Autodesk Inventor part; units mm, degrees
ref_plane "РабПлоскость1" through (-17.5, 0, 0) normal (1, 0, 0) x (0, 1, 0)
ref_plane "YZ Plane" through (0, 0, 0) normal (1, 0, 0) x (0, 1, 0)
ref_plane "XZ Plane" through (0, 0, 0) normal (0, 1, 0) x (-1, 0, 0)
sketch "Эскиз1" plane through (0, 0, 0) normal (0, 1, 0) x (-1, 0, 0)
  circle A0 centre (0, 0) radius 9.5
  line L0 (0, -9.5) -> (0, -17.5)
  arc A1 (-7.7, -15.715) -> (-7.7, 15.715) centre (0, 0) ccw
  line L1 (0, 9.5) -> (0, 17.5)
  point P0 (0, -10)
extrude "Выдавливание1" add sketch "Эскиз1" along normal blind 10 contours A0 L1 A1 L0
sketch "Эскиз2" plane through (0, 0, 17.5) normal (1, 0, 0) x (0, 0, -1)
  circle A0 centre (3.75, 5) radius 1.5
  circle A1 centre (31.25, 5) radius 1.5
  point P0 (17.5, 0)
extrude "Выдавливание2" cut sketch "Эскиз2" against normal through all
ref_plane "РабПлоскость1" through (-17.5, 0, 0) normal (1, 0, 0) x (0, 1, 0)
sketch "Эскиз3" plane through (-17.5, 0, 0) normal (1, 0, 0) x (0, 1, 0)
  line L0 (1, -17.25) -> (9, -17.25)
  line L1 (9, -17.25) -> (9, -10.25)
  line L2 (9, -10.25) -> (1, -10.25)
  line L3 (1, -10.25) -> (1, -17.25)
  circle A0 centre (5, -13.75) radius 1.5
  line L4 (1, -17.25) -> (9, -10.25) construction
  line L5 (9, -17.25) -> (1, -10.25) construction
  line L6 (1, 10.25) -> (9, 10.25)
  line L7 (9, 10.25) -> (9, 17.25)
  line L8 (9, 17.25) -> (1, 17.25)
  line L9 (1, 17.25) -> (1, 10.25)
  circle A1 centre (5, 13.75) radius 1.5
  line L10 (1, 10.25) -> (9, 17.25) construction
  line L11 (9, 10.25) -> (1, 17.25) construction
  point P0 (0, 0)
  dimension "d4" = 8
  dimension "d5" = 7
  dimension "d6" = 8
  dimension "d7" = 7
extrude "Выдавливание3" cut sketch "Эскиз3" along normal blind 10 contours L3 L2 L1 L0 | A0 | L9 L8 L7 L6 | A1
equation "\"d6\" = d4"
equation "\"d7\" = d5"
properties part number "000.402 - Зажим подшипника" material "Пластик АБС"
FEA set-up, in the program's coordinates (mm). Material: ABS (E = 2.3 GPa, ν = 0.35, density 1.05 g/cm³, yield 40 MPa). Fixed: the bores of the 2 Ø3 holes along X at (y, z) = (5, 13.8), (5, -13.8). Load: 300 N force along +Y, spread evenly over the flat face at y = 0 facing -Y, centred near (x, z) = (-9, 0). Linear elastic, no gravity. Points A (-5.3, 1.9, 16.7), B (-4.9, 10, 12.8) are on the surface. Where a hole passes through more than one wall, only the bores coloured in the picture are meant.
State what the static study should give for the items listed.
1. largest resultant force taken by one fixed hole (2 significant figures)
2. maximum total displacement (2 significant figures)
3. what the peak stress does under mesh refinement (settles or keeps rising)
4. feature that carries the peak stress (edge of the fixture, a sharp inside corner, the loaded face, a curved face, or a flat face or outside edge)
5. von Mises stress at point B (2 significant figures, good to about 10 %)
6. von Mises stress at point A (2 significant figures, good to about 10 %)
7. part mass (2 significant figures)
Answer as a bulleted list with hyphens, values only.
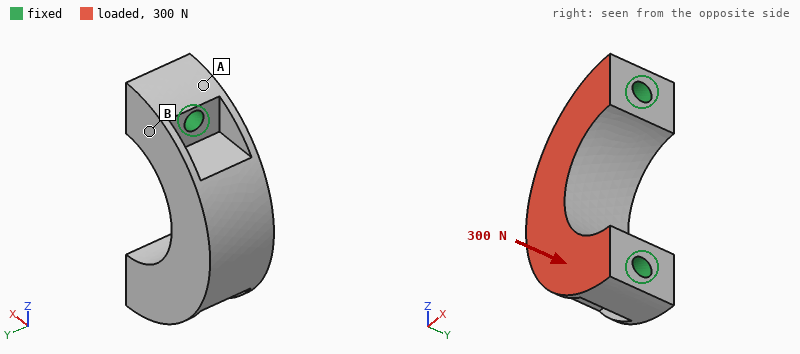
- 150 N
- 0.14 mm
- keeps rising
- edge of the fixture
- 6.4 MPa
- 2.4 MPa
- 3.1 g
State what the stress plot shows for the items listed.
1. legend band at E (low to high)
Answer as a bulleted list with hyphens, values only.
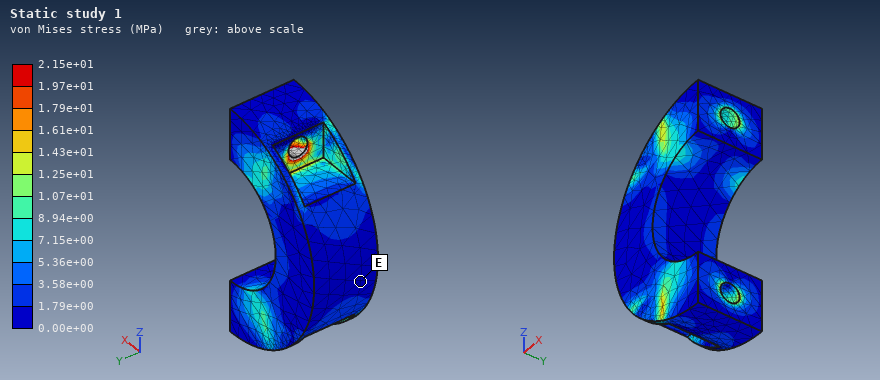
- 0.00e+00 to 1.79e+00 MPa
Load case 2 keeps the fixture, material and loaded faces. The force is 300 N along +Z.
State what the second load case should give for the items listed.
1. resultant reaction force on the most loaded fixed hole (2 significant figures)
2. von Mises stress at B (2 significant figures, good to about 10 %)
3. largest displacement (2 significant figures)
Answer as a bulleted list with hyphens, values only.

- 160 N
- 2.4 MPa
- 52 µm
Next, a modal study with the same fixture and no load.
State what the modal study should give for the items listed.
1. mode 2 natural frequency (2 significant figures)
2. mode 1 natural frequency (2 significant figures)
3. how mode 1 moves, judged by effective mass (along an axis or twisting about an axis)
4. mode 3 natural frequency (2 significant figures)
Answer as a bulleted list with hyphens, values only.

- 12 kHz
- 4900 Hz
- along Y
- 12 kHz
